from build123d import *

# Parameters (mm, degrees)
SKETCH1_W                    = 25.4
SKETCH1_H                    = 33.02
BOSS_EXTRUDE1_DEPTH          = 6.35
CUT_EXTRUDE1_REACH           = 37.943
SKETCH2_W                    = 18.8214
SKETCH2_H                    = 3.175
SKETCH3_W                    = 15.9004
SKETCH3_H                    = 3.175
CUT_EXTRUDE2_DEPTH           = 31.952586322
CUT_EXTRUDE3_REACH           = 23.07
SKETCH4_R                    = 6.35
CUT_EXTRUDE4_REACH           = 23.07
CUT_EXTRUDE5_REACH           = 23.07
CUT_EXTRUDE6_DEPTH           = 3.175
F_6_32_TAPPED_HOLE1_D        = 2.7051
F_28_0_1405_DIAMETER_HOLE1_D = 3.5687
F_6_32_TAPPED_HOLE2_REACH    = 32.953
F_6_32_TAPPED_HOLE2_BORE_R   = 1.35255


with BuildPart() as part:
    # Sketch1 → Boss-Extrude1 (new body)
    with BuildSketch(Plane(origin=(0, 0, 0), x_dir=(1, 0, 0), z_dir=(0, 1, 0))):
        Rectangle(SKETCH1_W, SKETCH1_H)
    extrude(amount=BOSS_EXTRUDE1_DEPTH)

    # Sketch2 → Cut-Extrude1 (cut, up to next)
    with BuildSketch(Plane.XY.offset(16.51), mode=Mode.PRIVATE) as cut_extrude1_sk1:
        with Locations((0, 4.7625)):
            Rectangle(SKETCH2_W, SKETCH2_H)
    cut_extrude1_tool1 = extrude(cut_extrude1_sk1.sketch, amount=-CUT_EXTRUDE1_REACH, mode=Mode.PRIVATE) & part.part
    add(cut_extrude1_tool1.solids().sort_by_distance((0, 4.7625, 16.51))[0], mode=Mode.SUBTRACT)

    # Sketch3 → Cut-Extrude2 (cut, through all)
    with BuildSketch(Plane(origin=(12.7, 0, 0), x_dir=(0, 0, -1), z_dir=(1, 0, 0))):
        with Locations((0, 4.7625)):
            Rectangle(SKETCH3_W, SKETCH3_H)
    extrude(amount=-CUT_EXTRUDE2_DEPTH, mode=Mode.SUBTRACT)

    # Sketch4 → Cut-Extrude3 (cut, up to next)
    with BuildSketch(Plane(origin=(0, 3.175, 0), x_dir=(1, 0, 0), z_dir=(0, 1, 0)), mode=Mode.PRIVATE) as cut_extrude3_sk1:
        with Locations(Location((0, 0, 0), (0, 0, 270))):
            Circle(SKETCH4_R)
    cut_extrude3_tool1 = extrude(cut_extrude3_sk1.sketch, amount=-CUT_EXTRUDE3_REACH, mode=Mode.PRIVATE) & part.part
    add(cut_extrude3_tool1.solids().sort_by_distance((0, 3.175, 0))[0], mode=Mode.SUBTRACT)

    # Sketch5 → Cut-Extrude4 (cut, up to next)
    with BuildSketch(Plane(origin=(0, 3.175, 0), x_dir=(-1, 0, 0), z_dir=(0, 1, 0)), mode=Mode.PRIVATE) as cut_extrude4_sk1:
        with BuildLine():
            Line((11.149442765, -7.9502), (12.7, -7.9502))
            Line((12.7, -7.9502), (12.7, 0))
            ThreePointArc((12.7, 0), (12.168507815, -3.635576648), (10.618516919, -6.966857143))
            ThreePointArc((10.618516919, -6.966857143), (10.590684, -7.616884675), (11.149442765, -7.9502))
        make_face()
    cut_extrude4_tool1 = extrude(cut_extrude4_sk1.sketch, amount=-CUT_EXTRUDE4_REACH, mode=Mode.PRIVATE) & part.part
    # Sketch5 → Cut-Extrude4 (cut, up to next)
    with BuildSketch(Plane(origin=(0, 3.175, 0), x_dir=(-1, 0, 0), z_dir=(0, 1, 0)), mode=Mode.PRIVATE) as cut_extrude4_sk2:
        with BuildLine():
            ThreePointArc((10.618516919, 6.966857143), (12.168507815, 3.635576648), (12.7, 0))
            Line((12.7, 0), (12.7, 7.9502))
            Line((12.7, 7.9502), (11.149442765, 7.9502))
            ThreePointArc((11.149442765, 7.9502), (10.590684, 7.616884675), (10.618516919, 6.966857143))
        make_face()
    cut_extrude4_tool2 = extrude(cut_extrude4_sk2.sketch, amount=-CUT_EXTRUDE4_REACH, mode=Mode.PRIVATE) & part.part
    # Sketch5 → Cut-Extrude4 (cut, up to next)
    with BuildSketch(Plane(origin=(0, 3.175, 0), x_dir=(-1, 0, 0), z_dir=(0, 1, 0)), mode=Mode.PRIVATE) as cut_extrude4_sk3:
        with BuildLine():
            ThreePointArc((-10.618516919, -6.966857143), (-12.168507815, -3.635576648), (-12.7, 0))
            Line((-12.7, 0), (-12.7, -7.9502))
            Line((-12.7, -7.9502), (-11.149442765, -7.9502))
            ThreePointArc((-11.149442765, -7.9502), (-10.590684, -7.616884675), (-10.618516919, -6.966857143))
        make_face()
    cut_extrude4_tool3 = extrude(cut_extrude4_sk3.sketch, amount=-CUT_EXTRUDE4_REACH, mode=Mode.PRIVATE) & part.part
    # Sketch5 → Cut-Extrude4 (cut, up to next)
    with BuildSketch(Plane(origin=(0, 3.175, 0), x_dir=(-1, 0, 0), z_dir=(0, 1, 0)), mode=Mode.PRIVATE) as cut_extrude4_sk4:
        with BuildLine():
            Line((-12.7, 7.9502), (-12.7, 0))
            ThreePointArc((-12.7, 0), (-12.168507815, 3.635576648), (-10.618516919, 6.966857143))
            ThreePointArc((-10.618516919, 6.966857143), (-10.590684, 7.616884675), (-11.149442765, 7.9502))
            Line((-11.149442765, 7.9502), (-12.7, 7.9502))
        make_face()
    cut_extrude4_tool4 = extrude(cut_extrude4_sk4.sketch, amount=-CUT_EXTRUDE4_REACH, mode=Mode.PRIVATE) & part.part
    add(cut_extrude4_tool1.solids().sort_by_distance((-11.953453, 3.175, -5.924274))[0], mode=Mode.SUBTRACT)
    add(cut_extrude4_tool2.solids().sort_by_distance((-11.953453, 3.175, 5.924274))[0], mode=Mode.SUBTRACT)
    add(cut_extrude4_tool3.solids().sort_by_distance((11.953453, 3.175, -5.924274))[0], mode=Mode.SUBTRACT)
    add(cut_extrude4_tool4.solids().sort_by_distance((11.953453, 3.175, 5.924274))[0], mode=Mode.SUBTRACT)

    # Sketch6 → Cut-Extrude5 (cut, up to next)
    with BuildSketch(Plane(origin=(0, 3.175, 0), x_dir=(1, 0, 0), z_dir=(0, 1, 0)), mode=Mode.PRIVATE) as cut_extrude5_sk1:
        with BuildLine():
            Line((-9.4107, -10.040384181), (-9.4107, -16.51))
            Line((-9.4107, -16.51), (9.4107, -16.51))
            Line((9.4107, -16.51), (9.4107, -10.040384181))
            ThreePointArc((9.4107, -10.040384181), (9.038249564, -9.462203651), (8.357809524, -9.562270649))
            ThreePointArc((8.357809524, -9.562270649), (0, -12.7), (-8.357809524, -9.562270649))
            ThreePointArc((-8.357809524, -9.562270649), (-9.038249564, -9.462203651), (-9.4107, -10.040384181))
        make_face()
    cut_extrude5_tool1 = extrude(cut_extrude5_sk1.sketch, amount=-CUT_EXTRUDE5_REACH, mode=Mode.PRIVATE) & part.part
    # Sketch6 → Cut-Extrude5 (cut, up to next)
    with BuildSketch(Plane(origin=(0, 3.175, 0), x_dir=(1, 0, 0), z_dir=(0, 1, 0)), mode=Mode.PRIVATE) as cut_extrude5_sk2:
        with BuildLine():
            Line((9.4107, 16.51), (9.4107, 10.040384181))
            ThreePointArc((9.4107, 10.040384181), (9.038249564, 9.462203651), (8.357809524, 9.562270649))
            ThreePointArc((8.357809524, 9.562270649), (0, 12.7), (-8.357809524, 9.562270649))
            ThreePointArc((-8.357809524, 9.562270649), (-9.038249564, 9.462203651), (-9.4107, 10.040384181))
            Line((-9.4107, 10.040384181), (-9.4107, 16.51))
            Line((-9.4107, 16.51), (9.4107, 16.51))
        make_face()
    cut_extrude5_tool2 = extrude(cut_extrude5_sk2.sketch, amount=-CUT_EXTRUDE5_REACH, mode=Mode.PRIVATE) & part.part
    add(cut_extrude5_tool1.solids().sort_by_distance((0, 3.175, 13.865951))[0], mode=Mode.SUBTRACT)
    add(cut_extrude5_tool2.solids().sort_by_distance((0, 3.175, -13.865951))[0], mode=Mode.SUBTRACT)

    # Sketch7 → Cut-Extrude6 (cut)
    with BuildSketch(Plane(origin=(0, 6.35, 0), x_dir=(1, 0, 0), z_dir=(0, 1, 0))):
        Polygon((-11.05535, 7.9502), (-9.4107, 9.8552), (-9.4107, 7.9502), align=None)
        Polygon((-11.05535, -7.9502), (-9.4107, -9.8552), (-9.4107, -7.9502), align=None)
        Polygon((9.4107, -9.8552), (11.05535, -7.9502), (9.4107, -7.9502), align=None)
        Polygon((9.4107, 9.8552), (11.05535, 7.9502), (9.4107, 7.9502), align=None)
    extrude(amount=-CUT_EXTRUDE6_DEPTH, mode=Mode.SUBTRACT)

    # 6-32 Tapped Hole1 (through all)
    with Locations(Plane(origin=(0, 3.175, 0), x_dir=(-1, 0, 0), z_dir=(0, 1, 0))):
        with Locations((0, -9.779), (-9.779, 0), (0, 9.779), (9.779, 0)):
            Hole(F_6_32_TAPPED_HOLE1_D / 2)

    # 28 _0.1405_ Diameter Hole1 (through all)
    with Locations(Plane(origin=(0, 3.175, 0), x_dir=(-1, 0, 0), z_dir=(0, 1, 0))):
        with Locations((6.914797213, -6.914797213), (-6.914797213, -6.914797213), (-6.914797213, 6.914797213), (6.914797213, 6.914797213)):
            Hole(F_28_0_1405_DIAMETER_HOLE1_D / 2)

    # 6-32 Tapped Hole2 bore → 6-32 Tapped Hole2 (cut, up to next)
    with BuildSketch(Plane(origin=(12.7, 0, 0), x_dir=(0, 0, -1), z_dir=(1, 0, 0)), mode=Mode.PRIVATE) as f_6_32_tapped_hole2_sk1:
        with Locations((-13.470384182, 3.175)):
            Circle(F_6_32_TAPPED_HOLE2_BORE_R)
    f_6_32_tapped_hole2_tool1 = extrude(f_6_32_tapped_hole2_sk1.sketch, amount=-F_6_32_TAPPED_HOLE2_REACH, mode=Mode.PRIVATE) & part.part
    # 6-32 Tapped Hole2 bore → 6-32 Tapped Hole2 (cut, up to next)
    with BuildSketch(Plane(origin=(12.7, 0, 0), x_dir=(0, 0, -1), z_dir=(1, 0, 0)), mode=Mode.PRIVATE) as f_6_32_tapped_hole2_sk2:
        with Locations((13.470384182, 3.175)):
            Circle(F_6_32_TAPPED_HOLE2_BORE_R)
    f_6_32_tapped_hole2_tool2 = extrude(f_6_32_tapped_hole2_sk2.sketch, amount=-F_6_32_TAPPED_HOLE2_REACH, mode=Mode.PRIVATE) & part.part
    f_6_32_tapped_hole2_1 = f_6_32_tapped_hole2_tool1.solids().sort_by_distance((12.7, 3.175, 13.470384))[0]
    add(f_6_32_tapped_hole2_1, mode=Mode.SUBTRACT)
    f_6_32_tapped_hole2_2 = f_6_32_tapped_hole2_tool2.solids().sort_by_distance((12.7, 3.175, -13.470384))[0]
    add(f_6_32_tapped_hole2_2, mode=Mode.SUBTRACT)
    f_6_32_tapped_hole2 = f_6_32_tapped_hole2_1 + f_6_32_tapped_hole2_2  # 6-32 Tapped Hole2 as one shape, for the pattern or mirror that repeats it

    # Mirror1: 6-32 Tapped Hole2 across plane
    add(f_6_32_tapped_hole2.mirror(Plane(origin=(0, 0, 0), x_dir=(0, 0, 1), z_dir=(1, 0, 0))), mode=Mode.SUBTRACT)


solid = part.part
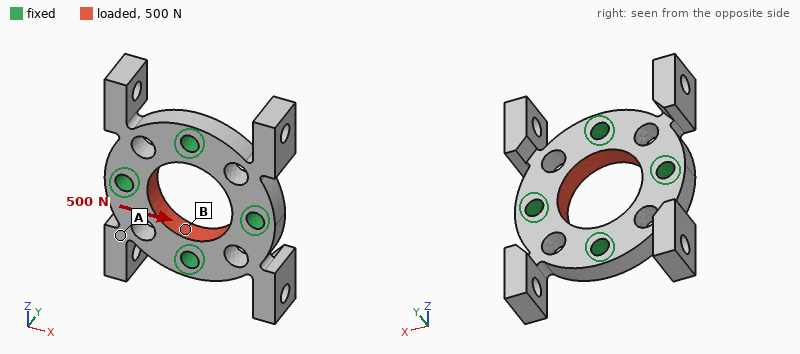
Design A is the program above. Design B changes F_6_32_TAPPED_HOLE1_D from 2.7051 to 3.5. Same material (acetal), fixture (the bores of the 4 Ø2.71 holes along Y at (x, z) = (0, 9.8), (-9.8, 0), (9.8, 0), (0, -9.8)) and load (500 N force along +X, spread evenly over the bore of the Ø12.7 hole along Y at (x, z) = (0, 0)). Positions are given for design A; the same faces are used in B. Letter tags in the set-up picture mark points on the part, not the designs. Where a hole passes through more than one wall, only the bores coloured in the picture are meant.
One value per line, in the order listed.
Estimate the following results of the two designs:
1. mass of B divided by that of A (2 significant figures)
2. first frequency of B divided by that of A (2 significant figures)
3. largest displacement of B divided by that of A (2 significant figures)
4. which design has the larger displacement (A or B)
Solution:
0.97
1.0
0.85
A
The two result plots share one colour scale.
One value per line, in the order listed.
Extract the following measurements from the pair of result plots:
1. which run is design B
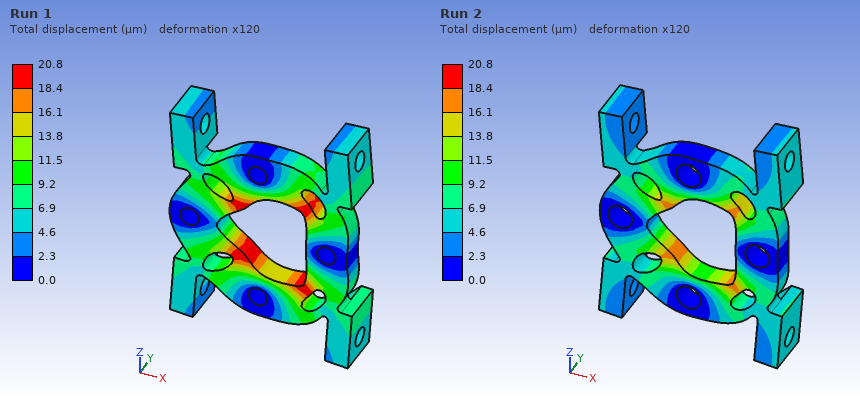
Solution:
Run 2
